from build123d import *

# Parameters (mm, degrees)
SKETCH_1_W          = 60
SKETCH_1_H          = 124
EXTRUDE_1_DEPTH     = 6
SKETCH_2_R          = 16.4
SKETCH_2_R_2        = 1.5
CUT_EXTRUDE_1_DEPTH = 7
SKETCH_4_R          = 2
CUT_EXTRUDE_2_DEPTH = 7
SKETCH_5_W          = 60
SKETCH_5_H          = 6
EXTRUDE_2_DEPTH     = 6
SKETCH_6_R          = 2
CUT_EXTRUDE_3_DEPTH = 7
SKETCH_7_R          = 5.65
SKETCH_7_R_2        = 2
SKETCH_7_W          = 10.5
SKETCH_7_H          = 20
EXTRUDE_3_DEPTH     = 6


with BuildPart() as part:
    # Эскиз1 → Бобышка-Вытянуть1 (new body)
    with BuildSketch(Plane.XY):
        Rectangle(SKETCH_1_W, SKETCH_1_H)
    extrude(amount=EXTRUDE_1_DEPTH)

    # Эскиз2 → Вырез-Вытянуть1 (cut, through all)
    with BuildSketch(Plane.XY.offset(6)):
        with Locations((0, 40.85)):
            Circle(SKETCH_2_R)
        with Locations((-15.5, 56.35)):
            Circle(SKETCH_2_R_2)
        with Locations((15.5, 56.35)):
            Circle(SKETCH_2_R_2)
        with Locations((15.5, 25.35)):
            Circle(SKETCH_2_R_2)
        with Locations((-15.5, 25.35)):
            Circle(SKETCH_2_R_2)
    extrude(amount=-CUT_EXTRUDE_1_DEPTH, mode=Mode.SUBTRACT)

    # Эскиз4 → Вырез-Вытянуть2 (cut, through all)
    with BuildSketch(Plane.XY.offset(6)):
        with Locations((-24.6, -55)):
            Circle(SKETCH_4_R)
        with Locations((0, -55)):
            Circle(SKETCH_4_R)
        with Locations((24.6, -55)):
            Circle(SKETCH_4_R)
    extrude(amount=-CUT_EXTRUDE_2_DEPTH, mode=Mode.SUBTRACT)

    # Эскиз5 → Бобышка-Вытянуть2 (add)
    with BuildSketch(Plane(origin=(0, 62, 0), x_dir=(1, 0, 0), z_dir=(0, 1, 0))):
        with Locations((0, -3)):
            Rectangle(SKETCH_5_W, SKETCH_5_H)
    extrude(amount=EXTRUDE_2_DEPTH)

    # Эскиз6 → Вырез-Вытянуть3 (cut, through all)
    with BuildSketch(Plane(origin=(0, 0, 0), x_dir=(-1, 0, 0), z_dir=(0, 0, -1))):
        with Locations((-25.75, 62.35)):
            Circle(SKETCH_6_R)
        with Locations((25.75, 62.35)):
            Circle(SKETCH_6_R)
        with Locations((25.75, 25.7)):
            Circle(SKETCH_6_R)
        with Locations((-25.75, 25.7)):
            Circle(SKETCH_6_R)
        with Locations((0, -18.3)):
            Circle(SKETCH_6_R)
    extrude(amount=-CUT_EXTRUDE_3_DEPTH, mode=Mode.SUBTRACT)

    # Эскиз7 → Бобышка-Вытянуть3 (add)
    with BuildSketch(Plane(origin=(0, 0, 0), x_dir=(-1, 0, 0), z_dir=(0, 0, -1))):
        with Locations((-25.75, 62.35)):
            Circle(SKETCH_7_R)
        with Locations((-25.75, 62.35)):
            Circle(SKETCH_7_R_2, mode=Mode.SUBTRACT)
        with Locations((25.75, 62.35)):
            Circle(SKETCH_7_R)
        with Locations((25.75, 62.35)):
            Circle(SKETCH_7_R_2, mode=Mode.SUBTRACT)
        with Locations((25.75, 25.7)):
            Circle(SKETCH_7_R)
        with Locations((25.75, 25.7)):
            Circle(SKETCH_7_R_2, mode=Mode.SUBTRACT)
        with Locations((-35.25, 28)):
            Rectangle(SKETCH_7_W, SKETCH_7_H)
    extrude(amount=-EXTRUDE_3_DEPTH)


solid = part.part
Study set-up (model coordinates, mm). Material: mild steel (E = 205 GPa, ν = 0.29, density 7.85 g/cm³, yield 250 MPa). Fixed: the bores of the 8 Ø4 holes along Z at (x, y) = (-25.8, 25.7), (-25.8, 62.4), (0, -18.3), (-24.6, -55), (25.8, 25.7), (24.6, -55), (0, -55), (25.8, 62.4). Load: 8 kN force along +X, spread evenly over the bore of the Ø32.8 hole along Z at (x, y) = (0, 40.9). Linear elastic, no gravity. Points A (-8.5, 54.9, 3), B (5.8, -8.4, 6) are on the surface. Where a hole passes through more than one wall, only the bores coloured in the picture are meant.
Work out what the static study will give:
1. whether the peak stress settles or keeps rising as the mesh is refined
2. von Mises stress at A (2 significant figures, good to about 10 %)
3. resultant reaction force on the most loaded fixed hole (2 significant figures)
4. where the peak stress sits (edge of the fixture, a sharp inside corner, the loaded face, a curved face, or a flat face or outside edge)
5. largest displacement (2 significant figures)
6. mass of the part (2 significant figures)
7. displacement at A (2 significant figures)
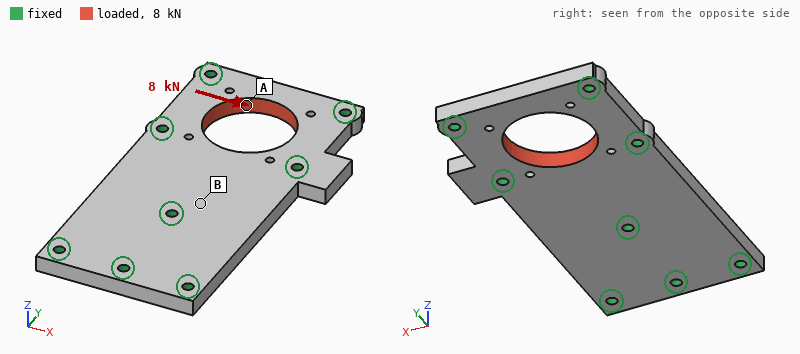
keeps rising
24 MPa
2.2 kN
edge of the fixture
3.2 µm
330 g
2.3 µm
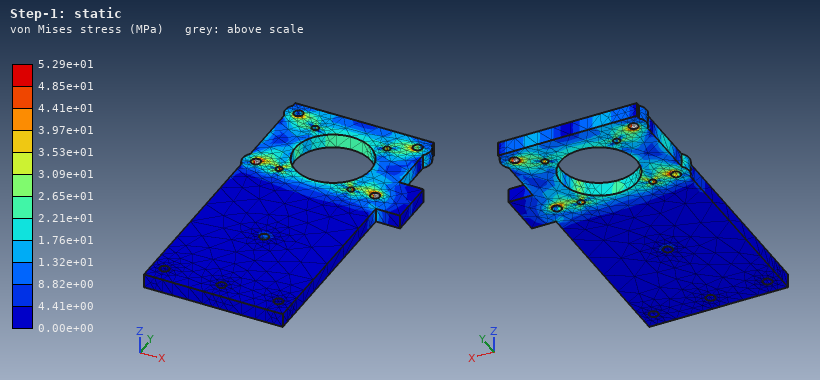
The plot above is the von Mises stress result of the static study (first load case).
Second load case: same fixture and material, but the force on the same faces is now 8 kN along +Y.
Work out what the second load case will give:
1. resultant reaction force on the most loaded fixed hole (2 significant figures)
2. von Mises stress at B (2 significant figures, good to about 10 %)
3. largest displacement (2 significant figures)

2.0 kN
6.9 MPa
7.0 µm
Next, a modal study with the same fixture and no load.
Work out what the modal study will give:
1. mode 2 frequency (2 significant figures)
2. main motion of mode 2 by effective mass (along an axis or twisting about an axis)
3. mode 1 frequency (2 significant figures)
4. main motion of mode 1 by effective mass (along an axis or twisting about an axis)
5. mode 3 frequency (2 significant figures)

8100 Hz
along Z
7300 Hz
twisting about Y
11 kHz
